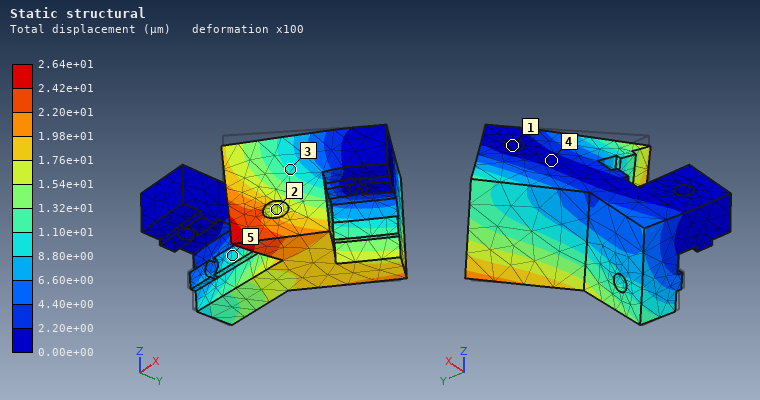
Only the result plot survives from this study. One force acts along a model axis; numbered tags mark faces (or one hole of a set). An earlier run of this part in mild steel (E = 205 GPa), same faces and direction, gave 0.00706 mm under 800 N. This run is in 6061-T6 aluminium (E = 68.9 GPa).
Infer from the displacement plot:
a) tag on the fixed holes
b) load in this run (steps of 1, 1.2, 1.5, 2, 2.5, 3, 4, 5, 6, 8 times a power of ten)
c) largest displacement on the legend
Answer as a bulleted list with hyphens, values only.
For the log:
- 1
- 1 kN
- 2.64e+01 µm
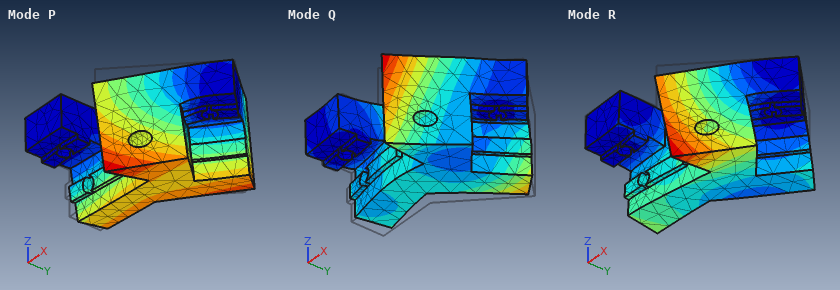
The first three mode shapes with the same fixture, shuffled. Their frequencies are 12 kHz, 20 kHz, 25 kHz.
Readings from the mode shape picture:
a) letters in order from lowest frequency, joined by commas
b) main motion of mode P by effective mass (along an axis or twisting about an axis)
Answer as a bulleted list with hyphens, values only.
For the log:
- P, R, Q
- along Y
